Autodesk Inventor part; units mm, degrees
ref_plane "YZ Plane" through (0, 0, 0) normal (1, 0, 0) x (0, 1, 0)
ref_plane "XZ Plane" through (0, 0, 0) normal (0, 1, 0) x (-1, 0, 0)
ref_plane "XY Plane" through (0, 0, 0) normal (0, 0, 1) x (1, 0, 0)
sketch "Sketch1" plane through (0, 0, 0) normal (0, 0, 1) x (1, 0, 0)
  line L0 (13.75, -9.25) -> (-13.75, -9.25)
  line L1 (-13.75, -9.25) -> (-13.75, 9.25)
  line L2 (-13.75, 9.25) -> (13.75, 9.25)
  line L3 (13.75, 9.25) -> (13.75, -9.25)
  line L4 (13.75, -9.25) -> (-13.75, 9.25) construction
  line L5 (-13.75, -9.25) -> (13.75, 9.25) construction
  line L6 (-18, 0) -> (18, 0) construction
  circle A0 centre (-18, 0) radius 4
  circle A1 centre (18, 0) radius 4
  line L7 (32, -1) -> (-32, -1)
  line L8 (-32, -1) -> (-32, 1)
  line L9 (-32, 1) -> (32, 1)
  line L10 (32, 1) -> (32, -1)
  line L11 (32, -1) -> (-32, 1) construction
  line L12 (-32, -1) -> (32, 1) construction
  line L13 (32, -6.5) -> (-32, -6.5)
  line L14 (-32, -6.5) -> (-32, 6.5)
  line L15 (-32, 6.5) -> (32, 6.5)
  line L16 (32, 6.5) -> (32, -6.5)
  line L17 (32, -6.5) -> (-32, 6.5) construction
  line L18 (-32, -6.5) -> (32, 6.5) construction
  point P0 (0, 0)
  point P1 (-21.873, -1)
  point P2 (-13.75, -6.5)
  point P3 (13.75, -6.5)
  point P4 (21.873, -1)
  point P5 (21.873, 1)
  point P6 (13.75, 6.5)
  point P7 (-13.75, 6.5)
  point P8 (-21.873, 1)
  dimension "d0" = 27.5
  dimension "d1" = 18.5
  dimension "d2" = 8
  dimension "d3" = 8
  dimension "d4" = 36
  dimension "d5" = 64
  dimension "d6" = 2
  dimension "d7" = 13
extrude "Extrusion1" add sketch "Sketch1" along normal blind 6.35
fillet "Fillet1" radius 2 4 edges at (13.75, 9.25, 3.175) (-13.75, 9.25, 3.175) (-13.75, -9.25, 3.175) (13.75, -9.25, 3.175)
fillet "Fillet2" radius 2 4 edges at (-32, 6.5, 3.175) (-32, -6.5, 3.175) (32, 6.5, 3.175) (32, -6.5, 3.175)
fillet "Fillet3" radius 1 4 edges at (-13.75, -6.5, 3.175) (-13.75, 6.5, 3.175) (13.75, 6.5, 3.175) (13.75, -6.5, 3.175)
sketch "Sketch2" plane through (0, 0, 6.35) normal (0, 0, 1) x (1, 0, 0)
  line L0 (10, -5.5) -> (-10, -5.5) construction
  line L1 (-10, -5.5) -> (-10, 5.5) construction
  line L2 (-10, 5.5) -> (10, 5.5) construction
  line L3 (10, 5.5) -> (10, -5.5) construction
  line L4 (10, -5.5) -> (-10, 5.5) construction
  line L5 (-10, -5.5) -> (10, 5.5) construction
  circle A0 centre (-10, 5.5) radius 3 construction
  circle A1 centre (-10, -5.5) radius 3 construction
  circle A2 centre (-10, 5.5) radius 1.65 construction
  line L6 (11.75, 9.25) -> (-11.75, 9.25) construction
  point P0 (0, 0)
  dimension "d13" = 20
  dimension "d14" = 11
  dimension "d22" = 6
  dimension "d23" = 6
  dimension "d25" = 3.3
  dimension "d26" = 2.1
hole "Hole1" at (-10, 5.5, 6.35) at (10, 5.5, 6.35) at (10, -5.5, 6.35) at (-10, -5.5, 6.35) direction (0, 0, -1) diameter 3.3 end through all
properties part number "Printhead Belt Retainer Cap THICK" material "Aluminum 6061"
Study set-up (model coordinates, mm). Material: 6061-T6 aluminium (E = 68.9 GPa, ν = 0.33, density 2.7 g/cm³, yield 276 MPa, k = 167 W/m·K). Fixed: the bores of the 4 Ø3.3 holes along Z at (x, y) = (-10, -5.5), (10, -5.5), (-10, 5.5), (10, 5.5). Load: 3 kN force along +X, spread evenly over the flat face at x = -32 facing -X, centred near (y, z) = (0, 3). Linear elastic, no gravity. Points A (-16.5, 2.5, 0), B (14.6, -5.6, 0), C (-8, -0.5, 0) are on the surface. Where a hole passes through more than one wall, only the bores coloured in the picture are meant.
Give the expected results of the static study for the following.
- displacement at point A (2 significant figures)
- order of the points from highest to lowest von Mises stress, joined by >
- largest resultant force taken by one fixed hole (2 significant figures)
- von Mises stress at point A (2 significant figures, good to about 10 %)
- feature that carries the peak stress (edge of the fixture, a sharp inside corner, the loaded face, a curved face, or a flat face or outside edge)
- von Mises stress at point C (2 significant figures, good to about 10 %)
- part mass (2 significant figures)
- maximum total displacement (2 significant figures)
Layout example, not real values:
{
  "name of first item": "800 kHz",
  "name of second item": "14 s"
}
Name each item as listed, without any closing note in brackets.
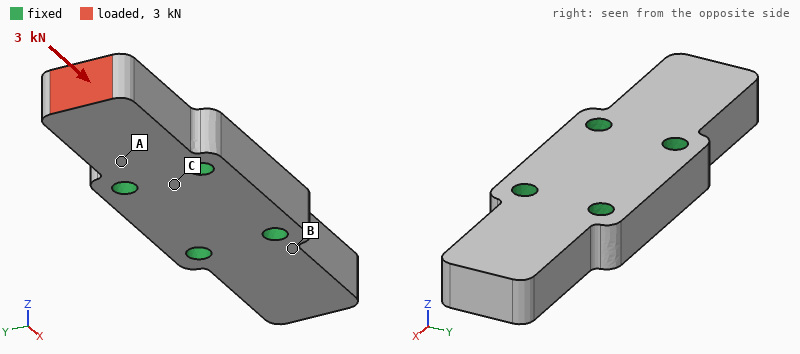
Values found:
{
  "displacement at point A": "3.2 µm",
  "order of the points from highest to lowest von Mises stress, joined by >": "A > C > B",
  "largest resultant force taken by one fixed hole": "1.5 kN",
  "von Mises stress at point A": "32 MPa",
  "feature that carries the peak stress": "a curved face",
  "von Mises stress at point C": "13 MPa",
  "part mass": "16 g",
  "maximum total displacement": "13 µm"
}
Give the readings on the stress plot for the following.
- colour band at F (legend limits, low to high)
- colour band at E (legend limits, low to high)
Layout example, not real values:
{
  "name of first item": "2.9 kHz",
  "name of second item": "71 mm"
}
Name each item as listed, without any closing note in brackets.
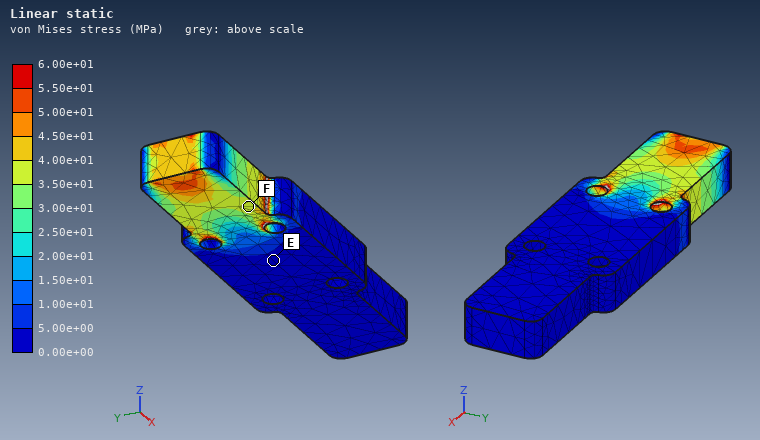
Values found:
{
  "colour band at F": "3.50e+01 to 4.00e+01 MPa",
  "colour band at E": "0.00e+00 to 5.00e+00 MPa"
}
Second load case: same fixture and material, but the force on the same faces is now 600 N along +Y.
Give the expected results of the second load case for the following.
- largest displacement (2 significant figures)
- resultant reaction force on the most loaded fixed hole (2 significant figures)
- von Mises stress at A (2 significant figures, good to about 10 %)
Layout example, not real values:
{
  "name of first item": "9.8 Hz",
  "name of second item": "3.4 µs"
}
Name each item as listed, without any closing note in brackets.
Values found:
{
  "largest displacement": "27 µm",
  "resultant reaction force on the most loaded fixed hole": "1.1 kN",
  "von Mises stress at A": "22 MPa"
}
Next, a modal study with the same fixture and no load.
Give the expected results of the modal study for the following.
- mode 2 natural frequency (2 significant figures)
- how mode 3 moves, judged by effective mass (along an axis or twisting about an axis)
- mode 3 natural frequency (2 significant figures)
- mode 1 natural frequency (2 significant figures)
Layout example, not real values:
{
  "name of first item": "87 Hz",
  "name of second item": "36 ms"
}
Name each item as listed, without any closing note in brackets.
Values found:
{
  "mode 2 natural frequency": "11 kHz",
  "how mode 3 moves, judged by effective mass": "along Y",
  "mode 3 natural frequency": "21 kHz",
  "mode 1 natural frequency": "11 kHz"
}
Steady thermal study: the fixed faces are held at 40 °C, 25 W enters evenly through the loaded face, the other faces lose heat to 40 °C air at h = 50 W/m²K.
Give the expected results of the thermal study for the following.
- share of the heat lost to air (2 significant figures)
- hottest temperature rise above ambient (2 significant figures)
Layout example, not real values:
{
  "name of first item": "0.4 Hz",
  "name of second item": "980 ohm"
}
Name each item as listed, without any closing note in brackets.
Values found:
{
  "share of the heat lost to air": "3.1 %",
  "hottest temperature rise above ambient": "40 K"
}
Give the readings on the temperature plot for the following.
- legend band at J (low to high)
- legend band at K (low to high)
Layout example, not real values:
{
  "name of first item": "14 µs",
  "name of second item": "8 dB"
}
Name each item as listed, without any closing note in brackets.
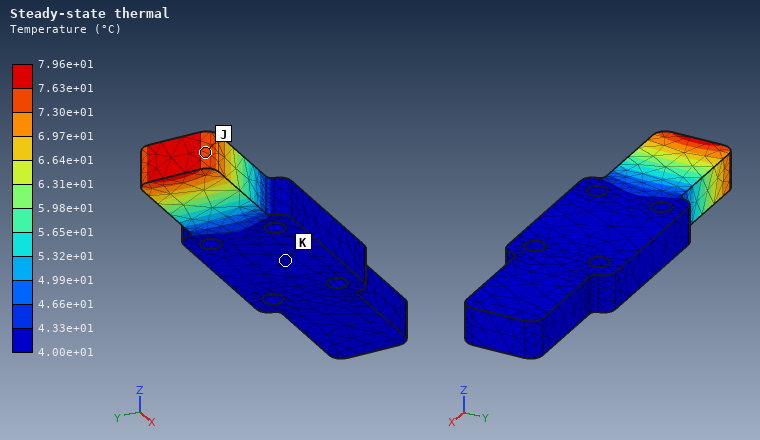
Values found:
{
  "legend band at J": "7.30e+01 to 7.63e+01 °C",
  "legend band at K": "4.00e+01 to 4.33e+01 °C"
}
